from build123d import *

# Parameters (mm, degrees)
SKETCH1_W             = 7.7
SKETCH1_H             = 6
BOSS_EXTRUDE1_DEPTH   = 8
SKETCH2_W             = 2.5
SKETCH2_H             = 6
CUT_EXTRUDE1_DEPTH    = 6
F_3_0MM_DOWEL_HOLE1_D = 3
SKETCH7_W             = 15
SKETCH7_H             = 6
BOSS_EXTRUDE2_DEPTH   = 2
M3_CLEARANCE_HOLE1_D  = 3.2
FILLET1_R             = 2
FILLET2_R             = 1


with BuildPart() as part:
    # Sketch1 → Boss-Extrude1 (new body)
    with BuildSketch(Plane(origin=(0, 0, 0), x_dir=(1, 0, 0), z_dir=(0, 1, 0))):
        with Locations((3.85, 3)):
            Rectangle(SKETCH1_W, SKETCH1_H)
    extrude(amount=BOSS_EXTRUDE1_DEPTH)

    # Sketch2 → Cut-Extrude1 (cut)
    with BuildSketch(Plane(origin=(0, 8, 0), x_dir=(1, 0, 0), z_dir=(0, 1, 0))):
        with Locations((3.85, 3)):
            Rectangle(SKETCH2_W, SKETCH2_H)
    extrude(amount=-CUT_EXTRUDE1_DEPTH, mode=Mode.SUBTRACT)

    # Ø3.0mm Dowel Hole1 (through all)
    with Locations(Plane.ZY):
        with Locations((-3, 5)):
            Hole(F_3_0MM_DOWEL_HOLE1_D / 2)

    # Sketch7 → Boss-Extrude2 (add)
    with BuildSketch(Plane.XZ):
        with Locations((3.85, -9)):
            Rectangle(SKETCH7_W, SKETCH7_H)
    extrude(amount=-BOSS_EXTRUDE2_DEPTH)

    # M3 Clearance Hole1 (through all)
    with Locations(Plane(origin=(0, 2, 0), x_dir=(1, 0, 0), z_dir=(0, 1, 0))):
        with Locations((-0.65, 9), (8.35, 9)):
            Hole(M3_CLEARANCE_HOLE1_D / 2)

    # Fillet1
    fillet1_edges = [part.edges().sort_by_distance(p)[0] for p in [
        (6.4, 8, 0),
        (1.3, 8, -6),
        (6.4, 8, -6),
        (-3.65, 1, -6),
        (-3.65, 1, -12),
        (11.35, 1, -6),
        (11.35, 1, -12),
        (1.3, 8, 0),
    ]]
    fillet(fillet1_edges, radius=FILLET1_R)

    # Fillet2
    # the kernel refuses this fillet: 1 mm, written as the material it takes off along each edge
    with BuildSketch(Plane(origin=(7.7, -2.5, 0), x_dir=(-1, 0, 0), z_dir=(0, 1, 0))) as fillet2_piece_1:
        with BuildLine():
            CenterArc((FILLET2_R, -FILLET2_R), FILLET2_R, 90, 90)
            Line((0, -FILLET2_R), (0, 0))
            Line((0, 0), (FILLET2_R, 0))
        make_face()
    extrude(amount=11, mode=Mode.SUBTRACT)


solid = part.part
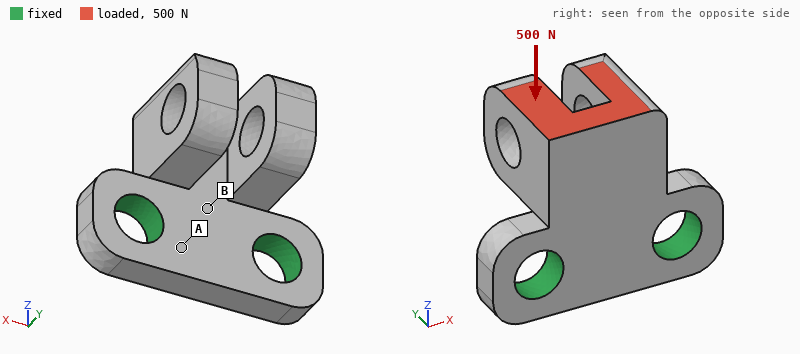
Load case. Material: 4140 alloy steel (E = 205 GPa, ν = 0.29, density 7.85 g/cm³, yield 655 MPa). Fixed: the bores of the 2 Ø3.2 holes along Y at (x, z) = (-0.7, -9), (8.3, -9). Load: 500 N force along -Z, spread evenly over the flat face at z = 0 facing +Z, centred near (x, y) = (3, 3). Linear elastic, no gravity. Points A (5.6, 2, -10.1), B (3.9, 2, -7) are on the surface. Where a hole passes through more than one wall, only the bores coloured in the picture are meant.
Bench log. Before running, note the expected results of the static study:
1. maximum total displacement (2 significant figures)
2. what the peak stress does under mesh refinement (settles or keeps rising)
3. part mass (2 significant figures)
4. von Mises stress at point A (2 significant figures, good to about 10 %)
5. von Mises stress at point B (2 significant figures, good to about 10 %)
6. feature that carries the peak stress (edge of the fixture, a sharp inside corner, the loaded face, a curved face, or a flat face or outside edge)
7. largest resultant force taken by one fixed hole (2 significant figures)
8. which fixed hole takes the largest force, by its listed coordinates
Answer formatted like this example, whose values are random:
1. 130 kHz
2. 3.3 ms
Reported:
1. 24 µm
2. keeps rising
3. 2.9 g
4. 28 MPa
5. 100 MPa
6. a sharp inside corner
7. 300 N
8. (-0.7, -9)
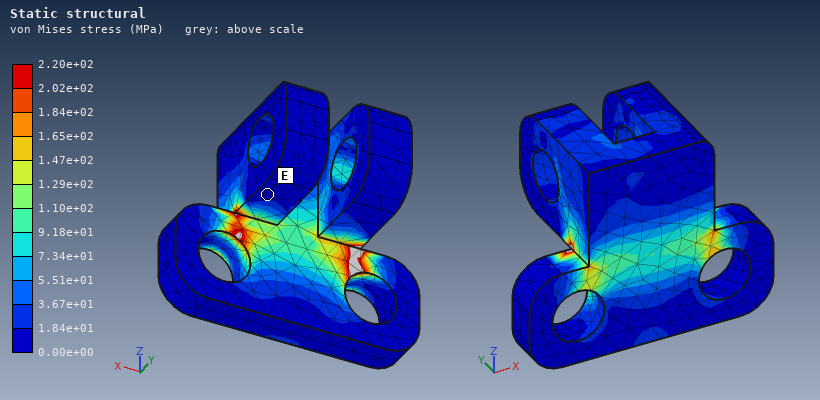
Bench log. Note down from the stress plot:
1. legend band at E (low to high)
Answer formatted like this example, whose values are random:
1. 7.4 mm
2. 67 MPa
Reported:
1. 0.00e+00 to 1.84e+01 MPa
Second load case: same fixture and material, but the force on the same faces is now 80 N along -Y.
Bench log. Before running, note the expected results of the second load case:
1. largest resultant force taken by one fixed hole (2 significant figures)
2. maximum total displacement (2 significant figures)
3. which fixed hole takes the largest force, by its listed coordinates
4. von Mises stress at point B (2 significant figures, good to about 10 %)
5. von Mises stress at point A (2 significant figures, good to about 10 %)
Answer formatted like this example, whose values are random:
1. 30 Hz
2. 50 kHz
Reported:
1. 47 N
2. 15 µm
3. (-0.7, -9)
4. 59 MPa
5. 13 MPa
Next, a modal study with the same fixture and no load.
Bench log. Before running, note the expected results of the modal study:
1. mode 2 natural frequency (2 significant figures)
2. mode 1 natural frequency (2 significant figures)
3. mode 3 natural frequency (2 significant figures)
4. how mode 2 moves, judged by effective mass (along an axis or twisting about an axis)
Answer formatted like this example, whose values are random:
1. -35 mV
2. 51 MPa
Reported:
1. 23 kHz
2. 13 kHz
3. 30 kHz
4. along X
